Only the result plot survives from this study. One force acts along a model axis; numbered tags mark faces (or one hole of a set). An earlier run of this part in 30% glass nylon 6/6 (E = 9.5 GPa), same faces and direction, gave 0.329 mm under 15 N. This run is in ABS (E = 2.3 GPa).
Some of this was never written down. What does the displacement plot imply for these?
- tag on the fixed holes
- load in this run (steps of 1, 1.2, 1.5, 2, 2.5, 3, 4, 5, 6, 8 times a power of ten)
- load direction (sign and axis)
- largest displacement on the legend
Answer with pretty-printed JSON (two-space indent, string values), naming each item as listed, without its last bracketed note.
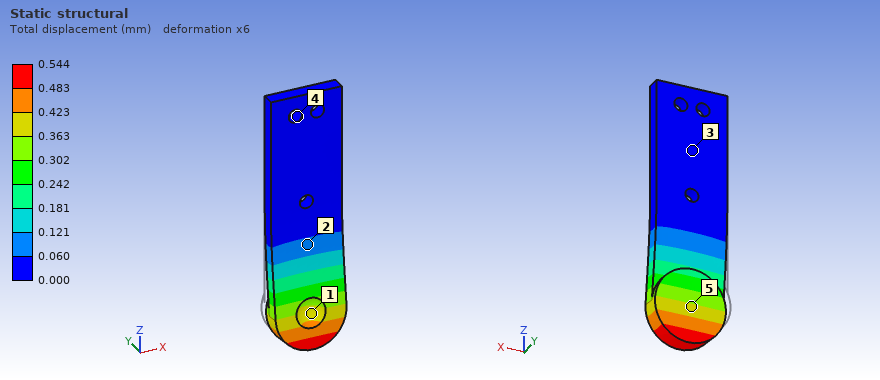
{
  "tag on the fixed holes": "4",
  "load in this run": "6 N",
  "load direction": "-Y",
  "largest displacement on the legend": "0.544 mm"
}
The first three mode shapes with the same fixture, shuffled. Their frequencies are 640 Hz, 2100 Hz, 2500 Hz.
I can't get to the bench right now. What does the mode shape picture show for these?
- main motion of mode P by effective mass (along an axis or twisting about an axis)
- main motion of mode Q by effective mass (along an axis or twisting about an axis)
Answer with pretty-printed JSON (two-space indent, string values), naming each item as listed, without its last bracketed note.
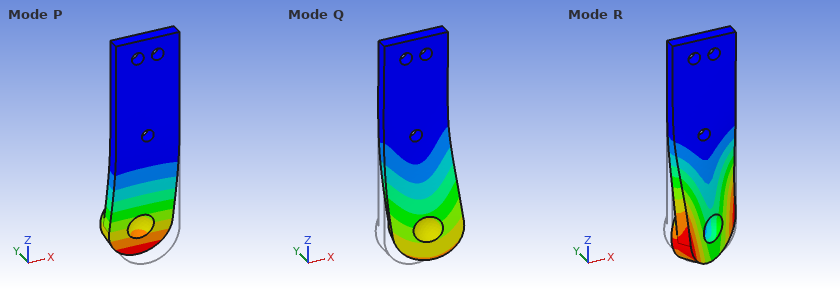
{
  "main motion of mode P by effective mass": "along Y",
  "main motion of mode Q by effective mass": "along X"
}
